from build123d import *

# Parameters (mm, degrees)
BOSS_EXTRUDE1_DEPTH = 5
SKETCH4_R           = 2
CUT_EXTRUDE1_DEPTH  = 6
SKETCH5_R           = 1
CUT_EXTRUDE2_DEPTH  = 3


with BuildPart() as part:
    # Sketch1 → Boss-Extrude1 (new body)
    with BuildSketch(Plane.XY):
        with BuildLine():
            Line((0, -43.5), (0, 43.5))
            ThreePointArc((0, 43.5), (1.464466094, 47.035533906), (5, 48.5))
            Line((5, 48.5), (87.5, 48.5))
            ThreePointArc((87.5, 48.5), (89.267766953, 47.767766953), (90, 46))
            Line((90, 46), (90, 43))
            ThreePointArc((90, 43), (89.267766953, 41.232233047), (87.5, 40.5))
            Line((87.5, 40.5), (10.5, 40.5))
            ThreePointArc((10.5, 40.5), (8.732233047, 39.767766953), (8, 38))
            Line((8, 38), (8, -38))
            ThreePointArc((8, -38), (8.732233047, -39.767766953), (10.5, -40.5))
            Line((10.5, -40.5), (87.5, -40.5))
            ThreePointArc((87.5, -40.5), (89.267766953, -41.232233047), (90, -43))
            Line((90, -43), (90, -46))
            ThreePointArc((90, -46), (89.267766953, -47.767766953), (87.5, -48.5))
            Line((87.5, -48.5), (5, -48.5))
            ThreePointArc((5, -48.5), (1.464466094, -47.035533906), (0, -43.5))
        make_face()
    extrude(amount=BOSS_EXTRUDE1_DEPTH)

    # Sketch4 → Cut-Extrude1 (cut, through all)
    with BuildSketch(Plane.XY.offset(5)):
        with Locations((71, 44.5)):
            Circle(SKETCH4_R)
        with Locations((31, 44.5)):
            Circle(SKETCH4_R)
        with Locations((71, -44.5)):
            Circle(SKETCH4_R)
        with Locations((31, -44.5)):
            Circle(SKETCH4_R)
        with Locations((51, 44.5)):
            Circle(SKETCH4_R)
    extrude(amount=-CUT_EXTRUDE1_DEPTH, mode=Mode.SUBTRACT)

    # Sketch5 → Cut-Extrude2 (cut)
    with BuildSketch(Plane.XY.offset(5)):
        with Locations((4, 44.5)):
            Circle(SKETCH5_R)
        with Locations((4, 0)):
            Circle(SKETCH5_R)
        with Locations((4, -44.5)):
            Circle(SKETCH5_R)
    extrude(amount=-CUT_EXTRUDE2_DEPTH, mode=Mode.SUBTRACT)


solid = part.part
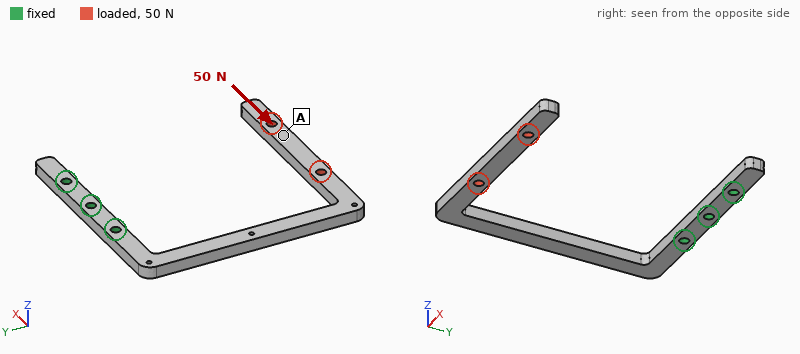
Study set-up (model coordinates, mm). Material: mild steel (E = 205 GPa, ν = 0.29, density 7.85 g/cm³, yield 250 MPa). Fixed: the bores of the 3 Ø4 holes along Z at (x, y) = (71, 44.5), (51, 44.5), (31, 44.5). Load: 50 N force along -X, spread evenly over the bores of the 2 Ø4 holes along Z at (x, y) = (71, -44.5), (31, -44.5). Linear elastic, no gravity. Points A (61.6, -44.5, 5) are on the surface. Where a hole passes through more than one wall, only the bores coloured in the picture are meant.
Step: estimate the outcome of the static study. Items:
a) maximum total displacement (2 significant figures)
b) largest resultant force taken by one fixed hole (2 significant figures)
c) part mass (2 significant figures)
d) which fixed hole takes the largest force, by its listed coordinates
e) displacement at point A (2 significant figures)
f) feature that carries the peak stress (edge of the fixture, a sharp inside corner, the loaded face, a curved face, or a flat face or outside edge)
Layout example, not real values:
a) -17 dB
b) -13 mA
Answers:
a) 0.75 mm
b) 62 N
c) 79 g
d) (31, 44.5)
e) 0.60 mm
f) a curved face
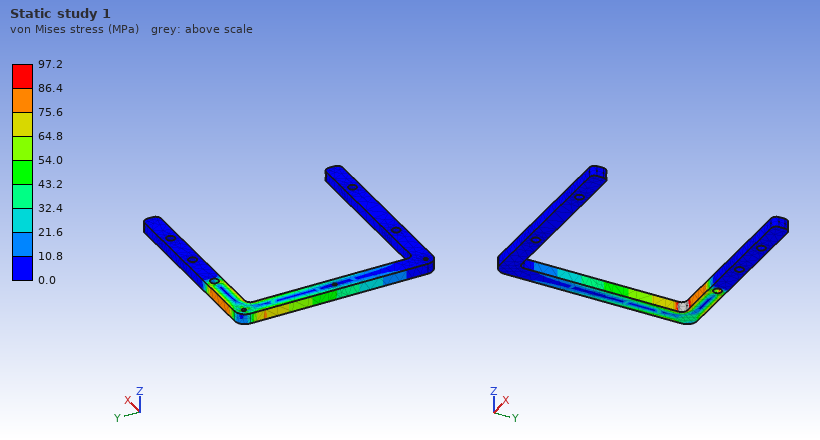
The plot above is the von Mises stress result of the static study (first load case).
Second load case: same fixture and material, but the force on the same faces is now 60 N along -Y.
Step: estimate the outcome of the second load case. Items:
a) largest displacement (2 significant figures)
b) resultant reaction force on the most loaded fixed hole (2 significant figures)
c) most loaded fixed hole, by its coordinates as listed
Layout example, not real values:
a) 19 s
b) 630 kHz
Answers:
a) 0.76 mm
b) 49 N
c) (31, 44.5)
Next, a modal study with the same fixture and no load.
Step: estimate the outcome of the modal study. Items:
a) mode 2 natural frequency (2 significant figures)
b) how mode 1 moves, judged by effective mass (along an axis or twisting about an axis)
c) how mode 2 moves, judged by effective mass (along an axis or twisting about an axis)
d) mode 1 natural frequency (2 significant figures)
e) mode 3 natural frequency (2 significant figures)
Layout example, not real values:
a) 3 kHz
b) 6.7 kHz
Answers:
a) 240 Hz
b) along Z
c) along X
d) 150 Hz
e) 390 Hz
